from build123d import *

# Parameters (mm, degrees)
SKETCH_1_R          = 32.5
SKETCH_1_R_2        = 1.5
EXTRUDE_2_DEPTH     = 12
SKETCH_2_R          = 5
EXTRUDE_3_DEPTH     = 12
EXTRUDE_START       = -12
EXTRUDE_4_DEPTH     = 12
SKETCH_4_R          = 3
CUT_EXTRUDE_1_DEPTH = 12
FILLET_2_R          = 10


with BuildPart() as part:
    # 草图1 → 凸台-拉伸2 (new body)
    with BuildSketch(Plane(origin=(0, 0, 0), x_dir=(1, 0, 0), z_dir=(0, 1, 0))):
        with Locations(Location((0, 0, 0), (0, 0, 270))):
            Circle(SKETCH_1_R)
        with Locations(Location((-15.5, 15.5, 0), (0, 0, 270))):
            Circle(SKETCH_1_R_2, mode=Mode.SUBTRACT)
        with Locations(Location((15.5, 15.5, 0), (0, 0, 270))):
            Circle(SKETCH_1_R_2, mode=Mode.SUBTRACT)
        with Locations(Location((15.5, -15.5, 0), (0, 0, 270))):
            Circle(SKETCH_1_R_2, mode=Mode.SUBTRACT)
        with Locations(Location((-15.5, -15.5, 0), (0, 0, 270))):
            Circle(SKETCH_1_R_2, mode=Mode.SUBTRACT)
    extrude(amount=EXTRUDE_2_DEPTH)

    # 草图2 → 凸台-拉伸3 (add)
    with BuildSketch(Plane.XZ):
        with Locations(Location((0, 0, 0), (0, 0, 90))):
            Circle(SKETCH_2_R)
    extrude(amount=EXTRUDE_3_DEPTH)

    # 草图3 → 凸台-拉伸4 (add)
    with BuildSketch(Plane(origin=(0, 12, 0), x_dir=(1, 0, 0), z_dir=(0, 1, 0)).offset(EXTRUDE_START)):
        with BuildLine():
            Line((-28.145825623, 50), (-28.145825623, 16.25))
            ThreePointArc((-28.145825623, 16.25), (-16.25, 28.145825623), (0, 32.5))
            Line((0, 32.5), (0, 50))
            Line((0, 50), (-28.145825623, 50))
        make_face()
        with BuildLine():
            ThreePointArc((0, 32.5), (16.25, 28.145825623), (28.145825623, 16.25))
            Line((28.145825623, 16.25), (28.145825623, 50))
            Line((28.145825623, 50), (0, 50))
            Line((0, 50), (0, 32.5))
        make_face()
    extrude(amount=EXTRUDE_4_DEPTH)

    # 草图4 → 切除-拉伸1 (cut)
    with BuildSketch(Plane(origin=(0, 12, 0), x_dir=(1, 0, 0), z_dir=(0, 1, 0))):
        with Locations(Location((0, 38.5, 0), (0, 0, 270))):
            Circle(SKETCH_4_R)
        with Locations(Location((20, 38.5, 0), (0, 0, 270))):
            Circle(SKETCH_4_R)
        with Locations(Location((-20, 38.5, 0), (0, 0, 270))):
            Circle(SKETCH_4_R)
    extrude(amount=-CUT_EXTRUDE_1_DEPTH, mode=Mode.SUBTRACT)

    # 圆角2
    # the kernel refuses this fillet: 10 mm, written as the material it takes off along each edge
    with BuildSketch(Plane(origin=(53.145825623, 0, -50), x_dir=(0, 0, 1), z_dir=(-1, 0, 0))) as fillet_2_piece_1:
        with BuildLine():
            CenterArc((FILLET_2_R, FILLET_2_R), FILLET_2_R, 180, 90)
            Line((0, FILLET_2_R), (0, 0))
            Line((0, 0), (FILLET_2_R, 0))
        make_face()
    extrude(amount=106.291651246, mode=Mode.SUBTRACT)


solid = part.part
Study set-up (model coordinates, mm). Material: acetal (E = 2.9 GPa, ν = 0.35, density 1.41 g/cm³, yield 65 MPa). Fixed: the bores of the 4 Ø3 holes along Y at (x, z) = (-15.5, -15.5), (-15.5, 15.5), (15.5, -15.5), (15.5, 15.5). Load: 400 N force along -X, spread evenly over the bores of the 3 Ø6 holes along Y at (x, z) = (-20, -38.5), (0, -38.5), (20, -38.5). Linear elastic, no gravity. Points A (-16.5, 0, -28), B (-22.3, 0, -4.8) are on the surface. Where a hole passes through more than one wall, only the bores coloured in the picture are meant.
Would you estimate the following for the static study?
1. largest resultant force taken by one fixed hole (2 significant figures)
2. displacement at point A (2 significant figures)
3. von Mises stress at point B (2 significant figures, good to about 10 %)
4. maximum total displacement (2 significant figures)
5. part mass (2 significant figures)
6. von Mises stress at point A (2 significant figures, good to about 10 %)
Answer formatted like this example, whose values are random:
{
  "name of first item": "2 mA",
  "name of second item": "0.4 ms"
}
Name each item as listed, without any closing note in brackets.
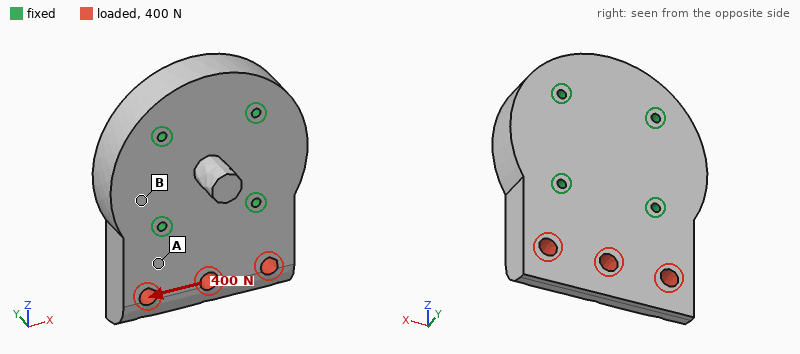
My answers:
{
  "largest resultant force taken by one fixed hole": "290 N",
  "displacement at point A": "13 µm",
  "von Mises stress at point B": "0.50 MPa",
  "maximum total displacement": "32 µm",
  "part mass": "75 g",
  "von Mises stress at point A": "1.2 MPa"
}
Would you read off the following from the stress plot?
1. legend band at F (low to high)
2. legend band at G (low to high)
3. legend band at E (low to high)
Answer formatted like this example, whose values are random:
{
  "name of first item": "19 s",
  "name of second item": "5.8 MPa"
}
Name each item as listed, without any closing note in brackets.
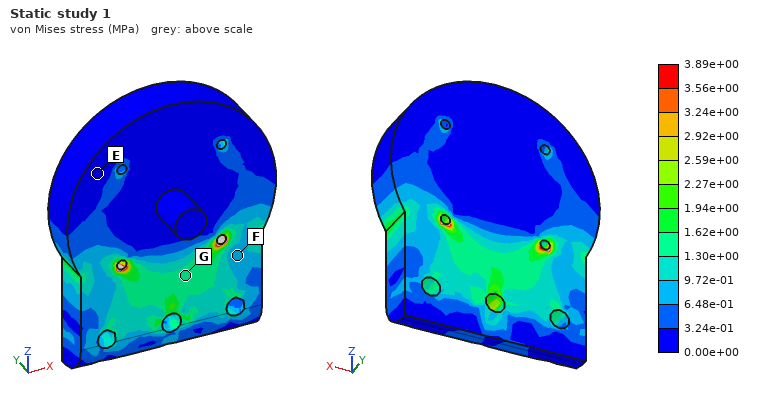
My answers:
{
  "legend band at F": "6.48e-01 to 9.72e-01 MPa",
  "legend band at G": "1.30e+00 to 1.62e+00 MPa",
  "legend band at E": "0.00e+00 to 3.24e-01 MPa"
}
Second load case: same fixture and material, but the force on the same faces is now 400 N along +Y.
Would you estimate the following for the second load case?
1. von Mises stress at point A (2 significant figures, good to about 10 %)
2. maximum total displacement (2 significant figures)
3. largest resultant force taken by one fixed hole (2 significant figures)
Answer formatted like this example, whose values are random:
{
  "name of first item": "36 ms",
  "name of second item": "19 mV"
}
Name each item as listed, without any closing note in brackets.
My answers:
{
  "von Mises stress at point A": "3.1 MPa",
  "maximum total displacement": "0.19 mm",
  "largest resultant force taken by one fixed hole": "270 N"
}
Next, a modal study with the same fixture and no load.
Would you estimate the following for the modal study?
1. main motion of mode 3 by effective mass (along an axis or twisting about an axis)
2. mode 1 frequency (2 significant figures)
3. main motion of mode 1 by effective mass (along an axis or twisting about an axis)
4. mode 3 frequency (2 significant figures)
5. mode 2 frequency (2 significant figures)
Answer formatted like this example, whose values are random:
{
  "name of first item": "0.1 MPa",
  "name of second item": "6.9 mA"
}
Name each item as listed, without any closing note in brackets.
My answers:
{
  "main motion of mode 3 by effective mass": "along X",
  "mode 1 frequency": "2100 Hz",
  "main motion of mode 1 by effective mass": "along Y",
  "mode 3 frequency": "4500 Hz",
  "mode 2 frequency": "3200 Hz"
}
